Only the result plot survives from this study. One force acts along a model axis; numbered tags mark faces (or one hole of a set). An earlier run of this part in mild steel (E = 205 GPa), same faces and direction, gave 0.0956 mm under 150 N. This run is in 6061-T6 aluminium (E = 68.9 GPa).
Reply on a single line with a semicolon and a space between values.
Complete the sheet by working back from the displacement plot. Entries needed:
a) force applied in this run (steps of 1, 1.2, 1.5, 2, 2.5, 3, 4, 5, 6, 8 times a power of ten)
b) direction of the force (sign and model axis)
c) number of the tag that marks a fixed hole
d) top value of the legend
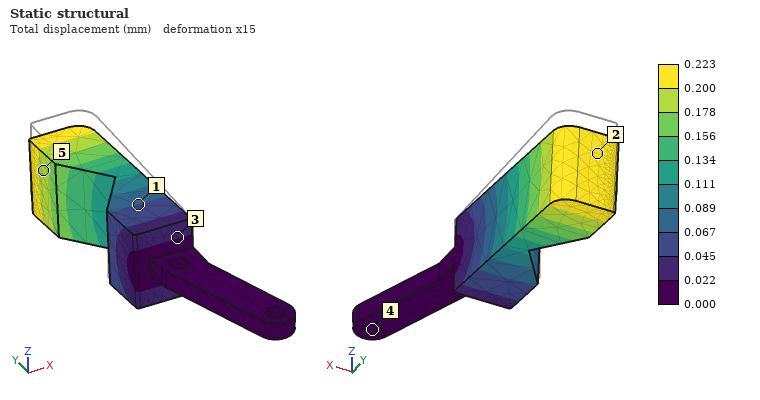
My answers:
120 N; -Z; 4; 0.223 mm
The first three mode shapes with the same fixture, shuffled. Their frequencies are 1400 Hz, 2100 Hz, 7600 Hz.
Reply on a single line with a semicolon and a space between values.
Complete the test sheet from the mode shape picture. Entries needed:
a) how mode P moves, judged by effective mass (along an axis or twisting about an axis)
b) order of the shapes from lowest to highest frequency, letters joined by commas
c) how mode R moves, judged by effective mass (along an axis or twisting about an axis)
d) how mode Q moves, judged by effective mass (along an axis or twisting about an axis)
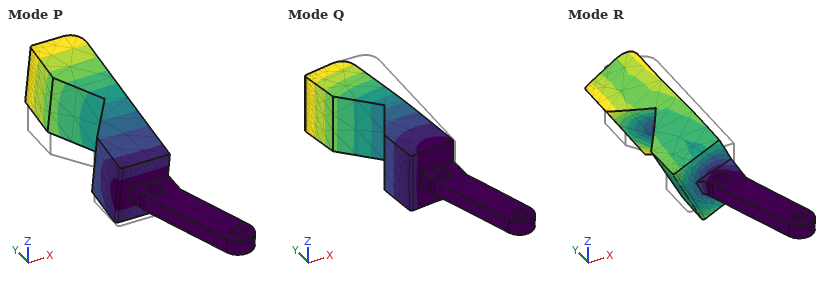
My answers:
along Z; P, Q, R; twisting about Y; along X
